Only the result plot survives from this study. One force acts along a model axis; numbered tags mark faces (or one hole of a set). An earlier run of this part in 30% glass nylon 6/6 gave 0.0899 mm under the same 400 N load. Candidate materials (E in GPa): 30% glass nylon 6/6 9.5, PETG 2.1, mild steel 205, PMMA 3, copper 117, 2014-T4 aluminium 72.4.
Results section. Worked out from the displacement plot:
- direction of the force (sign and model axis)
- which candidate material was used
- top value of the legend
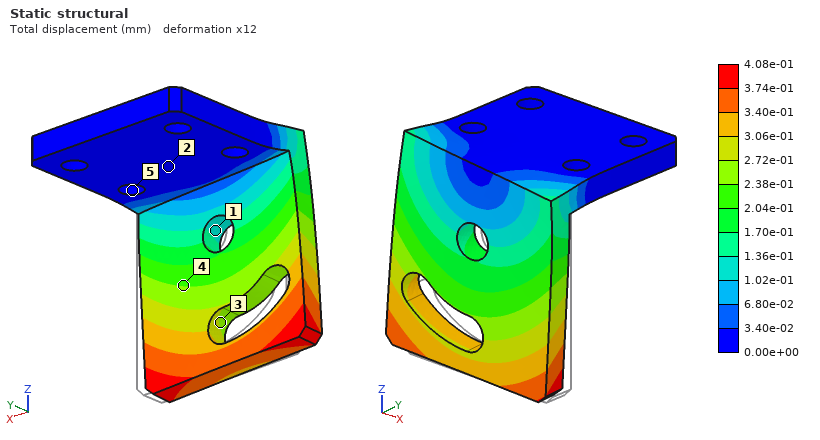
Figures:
-X
PETG
4.08e-01 mm
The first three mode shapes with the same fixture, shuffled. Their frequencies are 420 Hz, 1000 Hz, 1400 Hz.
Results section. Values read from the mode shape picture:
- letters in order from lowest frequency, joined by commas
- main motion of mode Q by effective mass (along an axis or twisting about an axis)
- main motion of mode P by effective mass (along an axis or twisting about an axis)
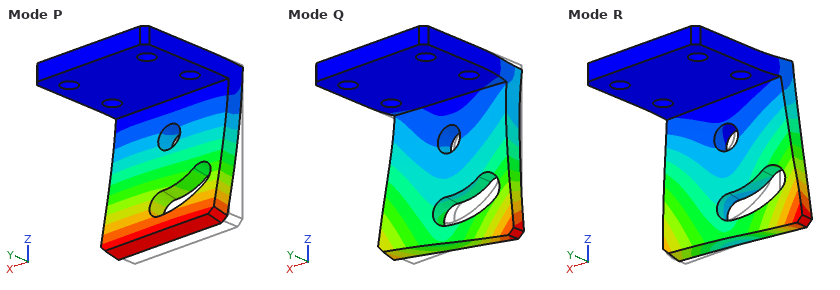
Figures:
P, R, Q
along X
along Y
